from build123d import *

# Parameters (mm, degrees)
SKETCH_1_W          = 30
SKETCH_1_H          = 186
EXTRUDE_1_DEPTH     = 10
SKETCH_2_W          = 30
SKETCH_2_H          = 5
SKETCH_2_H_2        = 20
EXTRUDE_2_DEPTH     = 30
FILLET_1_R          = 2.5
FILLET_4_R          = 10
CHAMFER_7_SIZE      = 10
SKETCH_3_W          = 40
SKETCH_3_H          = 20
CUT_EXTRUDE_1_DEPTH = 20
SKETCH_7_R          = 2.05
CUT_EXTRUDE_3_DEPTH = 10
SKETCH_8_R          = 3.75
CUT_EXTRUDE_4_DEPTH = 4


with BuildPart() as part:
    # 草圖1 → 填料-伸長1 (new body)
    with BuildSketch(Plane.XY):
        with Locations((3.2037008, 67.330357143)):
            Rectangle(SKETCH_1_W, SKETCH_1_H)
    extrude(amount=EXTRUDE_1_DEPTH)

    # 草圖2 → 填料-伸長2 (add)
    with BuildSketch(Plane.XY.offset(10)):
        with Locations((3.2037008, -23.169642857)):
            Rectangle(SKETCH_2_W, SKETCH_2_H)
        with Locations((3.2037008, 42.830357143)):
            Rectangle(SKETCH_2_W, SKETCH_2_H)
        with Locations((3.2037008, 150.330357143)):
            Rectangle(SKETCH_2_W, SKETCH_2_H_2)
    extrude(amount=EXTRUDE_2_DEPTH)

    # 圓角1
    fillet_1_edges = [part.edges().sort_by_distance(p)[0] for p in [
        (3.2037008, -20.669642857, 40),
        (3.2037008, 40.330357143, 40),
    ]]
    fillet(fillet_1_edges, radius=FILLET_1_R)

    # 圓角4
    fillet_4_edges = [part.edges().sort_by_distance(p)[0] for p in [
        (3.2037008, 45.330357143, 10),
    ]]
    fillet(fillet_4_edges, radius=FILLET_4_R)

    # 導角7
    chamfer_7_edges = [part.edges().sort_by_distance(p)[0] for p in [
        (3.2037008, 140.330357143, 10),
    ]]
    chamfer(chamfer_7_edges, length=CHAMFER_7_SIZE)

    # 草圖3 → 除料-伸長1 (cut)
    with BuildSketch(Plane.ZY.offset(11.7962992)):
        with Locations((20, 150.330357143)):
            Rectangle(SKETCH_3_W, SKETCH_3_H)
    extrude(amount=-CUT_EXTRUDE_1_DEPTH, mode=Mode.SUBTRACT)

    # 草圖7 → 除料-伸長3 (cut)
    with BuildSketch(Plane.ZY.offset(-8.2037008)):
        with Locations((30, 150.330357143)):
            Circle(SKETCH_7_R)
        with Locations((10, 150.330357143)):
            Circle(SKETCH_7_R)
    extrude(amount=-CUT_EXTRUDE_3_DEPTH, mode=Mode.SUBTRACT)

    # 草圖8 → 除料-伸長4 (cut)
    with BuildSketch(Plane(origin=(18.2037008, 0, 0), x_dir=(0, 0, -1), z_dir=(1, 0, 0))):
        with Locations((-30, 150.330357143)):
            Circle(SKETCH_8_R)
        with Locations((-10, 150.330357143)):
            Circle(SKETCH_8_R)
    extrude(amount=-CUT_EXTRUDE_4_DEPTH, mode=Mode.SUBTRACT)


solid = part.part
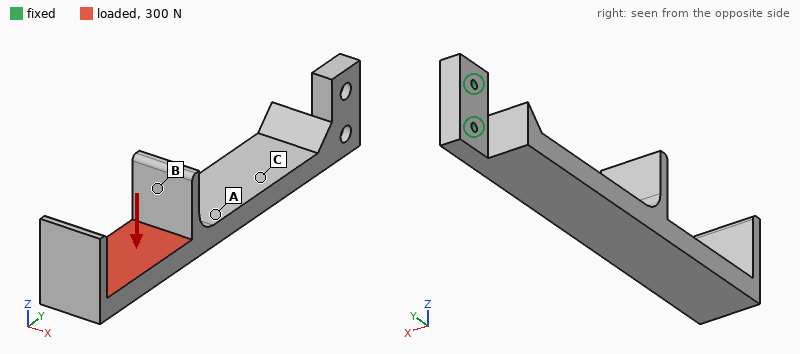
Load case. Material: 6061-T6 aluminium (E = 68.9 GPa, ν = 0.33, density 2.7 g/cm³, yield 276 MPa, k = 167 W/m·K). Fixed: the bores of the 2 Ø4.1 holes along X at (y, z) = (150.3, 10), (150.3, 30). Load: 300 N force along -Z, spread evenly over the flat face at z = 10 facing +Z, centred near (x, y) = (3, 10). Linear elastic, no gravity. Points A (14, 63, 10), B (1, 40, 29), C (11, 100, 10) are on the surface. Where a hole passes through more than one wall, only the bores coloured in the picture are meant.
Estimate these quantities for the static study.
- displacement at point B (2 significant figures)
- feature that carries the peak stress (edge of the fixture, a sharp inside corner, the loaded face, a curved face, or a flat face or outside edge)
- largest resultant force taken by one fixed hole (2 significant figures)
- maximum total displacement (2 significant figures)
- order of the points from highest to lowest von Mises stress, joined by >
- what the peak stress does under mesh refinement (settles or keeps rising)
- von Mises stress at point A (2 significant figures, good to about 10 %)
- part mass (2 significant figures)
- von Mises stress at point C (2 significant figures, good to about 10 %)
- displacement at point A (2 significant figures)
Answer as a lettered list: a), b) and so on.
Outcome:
a) 1.1 mm
b) edge of the fixture
c) 2.0 kN
d) 2.2 mm
e) C > A > B
f) keeps rising
g) 32 MPa
h) 180 g
i) 54 MPa
j) 0.68 mm
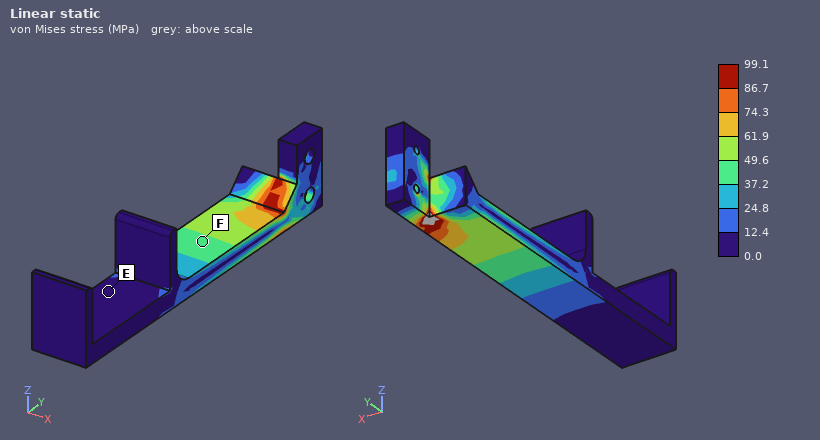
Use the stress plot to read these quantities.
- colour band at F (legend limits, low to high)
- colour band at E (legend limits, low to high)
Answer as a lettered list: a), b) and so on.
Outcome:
a) 37.2 to 49.6 MPa
b) 0.0 to 12.4 MPa
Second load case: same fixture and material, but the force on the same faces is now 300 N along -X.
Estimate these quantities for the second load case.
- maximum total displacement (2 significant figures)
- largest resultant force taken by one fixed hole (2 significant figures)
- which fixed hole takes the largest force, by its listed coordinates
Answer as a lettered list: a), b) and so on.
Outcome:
a) 1.7 mm
b) 410 N
c) (150.3, 10)
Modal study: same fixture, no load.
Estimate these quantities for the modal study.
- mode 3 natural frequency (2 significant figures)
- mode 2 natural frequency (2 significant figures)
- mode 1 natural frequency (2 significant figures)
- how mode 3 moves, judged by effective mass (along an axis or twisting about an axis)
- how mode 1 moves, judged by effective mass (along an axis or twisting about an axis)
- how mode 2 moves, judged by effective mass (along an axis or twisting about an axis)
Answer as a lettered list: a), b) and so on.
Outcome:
a) 1300 Hz
b) 240 Hz
c) 230 Hz
d) along Z
e) along Z
f) along X
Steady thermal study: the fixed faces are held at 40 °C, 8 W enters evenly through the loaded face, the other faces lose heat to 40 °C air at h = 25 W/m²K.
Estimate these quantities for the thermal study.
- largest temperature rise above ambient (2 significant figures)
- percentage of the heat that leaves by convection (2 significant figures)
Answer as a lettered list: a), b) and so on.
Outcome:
a) 14 K
b) 48 %
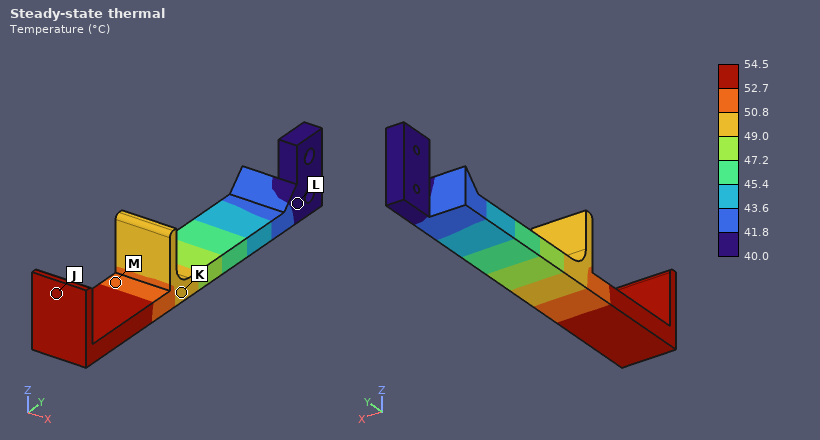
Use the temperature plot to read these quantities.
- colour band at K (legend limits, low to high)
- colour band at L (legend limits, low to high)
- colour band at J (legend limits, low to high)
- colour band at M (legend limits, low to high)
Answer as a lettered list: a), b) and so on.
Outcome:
a) 49.0 to 50.8 °C
b) 40.0 to 41.8 °C
c) 52.7 to 54.5 °C
d) 50.8 to 52.7 °C
